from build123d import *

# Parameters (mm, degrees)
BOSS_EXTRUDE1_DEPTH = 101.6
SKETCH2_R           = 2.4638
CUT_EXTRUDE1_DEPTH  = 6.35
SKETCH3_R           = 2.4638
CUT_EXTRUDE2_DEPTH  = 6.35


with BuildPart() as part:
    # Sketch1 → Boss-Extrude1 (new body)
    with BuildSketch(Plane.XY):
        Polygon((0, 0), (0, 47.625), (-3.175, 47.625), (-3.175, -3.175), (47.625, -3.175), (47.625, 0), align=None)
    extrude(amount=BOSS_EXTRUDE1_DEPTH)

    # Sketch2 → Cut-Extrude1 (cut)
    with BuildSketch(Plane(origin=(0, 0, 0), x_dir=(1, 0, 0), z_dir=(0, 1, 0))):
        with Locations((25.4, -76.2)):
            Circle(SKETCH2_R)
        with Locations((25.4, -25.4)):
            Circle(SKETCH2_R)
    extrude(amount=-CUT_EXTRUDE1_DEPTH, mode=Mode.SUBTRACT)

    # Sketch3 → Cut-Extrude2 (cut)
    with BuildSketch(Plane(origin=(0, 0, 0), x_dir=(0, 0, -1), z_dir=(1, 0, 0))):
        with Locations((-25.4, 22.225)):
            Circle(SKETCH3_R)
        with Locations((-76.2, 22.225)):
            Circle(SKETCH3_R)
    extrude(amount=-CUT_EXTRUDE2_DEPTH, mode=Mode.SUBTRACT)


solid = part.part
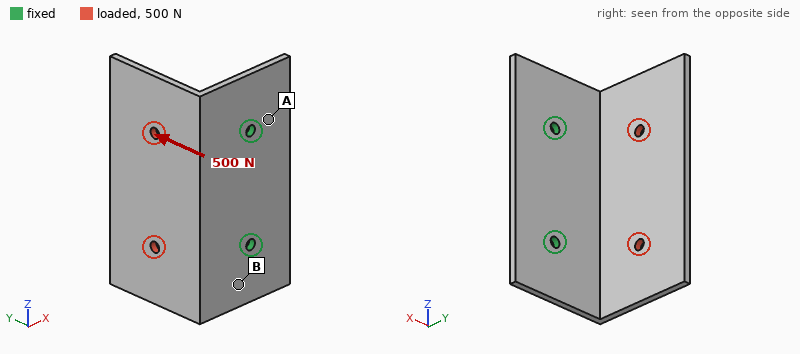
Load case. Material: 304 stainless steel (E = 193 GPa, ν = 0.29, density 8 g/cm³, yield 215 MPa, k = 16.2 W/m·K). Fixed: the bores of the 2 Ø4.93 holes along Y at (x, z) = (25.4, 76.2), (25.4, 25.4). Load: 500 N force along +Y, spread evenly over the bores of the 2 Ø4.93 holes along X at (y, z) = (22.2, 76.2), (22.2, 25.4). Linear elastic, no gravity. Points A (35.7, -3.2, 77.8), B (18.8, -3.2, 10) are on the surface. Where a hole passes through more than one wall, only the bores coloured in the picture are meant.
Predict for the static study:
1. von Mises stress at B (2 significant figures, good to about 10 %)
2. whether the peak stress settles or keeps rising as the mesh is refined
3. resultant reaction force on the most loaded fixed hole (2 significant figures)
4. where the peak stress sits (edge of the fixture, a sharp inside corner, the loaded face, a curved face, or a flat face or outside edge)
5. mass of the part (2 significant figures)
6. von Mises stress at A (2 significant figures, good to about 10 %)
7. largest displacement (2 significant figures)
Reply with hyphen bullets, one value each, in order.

- 43 MPa
- keeps rising
- 250 N
- edge of the fixture
- 250 g
- 16 MPa
- 0.22 mm
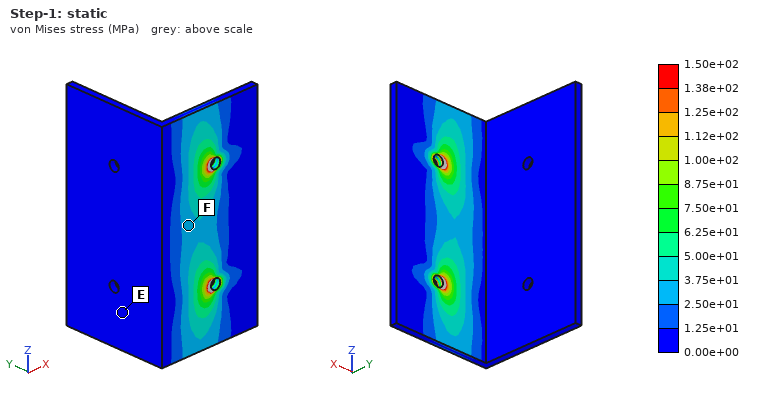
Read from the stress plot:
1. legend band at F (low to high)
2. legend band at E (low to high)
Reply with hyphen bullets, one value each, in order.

- 2.50e+01 to 3.75e+01 MPa
- 0.00e+00 to 1.25e+01 MPa
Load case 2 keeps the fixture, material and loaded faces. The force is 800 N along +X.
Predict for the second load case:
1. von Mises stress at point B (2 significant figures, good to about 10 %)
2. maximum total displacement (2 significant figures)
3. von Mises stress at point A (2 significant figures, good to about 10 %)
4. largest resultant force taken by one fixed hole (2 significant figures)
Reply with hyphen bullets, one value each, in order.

- 88 MPa
- 0.69 mm
- 37 MPa
- 400 N
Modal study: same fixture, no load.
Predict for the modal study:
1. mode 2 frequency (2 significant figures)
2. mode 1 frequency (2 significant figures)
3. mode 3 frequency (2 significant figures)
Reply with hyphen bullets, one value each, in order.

- 930 Hz
- 530 Hz
- 1500 Hz
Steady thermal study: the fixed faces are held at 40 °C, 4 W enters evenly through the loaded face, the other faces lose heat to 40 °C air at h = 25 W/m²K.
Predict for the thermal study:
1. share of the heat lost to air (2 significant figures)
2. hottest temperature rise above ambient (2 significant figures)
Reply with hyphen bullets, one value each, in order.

- 83 %
- 22 K
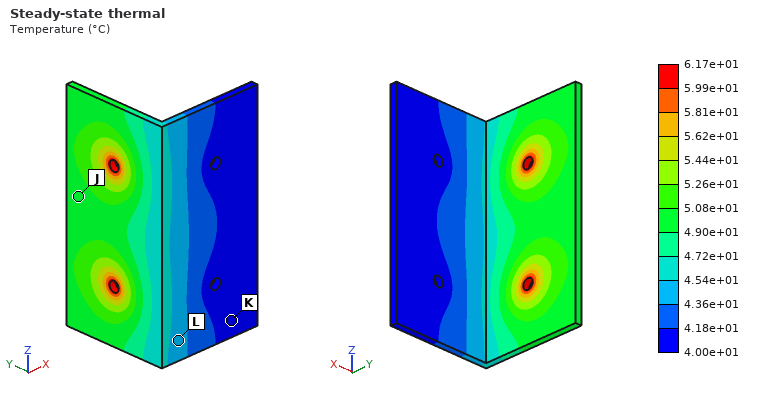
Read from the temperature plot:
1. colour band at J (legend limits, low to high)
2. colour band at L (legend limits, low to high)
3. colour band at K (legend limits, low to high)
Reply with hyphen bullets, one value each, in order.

- 4.90e+01 to 5.08e+01 °C
- 4.36e+01 to 4.54e+01 °C
- 4.00e+01 to 4.18e+01 °C
